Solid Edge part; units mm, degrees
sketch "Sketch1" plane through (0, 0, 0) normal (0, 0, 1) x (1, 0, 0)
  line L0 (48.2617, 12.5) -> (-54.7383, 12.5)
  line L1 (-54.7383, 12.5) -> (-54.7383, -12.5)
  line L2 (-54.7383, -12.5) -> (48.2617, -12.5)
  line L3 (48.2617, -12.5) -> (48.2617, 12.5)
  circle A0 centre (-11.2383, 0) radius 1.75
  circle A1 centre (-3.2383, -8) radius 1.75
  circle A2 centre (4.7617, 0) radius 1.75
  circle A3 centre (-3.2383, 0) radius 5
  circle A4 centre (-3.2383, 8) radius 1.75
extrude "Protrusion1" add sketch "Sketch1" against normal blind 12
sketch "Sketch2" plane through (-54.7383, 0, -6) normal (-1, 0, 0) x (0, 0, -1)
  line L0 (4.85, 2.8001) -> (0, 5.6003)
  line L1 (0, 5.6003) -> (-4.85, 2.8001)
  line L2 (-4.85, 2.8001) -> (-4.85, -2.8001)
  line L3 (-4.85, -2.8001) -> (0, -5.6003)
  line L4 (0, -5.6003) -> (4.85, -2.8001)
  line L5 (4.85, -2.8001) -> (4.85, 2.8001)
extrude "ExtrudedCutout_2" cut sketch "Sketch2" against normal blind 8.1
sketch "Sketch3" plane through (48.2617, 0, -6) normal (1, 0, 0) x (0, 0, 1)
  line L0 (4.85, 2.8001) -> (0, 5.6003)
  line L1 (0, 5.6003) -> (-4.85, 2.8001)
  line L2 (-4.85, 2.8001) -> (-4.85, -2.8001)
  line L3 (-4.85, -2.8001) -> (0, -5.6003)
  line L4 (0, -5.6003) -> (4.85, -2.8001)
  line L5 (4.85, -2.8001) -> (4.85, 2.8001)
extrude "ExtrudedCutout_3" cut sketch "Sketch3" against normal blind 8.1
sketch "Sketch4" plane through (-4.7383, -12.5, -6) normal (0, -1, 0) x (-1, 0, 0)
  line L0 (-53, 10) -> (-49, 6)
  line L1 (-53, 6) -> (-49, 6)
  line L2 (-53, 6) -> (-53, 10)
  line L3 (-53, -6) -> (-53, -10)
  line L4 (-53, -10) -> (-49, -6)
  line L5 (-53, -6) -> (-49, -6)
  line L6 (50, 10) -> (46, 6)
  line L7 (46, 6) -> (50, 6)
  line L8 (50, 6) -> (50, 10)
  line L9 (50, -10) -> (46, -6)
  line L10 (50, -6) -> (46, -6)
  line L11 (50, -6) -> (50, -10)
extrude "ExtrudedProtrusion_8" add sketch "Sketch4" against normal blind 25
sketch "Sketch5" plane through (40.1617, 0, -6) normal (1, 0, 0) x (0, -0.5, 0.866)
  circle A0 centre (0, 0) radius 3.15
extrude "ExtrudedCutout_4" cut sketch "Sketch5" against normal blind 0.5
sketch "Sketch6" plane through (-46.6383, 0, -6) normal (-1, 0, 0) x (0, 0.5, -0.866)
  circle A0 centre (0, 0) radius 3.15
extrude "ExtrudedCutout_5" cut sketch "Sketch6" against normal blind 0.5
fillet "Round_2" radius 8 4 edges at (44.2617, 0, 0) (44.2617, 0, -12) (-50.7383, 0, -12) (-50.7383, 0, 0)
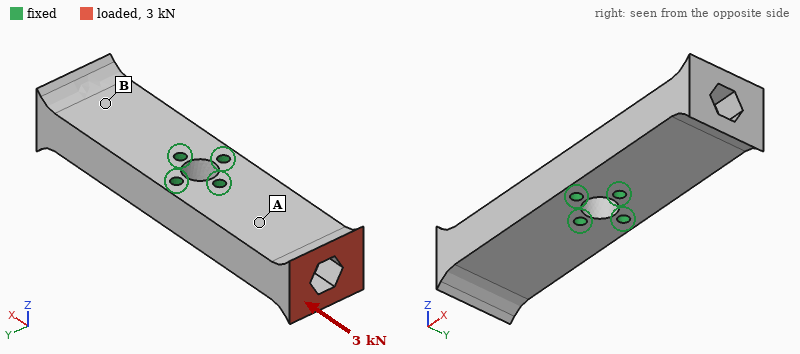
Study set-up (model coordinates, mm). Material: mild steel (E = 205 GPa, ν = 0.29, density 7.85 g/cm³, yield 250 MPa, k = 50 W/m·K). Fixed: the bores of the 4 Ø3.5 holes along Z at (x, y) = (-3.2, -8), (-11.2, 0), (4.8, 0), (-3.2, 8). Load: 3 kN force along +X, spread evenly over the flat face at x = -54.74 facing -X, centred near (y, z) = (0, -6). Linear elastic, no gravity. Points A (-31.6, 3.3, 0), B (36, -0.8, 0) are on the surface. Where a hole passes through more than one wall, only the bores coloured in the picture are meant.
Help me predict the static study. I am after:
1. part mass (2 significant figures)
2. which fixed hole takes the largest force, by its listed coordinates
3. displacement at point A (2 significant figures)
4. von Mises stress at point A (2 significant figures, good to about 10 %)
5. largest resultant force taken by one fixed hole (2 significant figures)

230 g
(-11.2, 0)
1.2 µm
9.9 MPa
1.6 kN
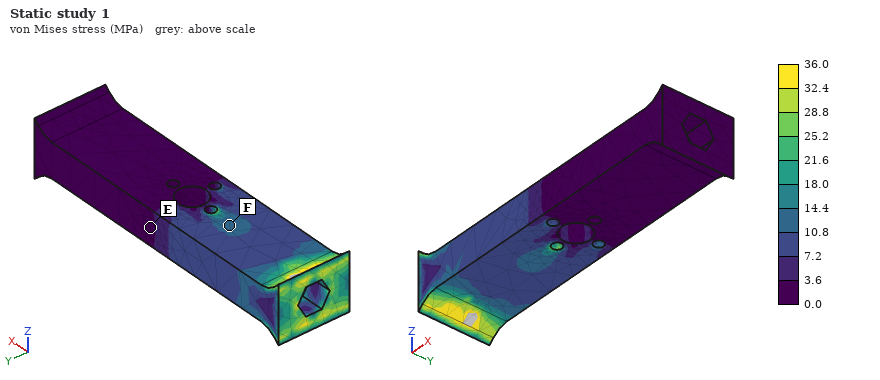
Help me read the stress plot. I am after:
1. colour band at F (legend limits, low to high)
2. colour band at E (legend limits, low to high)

10.8 to 14.4 MPa
0.0 to 3.6 MPa
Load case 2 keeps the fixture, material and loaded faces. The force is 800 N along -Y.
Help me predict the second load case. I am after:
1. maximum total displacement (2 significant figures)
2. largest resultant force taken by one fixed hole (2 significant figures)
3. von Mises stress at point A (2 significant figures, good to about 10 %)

13 µm
1.7 kN
7.7 MPa
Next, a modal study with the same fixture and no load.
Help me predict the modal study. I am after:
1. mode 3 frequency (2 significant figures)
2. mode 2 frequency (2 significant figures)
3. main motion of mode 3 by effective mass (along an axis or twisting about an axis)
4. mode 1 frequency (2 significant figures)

7300 Hz
4600 Hz
twisting about Z
4600 Hz
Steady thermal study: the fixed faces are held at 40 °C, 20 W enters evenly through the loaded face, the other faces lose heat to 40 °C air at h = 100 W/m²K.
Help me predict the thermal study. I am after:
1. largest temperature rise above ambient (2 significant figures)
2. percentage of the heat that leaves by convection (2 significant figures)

48 K
42 %
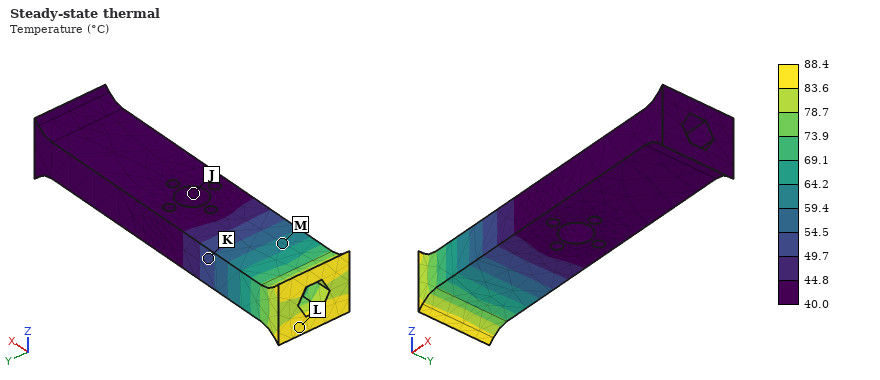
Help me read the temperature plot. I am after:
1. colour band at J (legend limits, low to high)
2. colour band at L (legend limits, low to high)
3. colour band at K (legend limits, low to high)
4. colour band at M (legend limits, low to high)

40.0 to 44.8 °C
83.6 to 88.4 °C
49.7 to 54.5 °C
59.4 to 64.2 °C
